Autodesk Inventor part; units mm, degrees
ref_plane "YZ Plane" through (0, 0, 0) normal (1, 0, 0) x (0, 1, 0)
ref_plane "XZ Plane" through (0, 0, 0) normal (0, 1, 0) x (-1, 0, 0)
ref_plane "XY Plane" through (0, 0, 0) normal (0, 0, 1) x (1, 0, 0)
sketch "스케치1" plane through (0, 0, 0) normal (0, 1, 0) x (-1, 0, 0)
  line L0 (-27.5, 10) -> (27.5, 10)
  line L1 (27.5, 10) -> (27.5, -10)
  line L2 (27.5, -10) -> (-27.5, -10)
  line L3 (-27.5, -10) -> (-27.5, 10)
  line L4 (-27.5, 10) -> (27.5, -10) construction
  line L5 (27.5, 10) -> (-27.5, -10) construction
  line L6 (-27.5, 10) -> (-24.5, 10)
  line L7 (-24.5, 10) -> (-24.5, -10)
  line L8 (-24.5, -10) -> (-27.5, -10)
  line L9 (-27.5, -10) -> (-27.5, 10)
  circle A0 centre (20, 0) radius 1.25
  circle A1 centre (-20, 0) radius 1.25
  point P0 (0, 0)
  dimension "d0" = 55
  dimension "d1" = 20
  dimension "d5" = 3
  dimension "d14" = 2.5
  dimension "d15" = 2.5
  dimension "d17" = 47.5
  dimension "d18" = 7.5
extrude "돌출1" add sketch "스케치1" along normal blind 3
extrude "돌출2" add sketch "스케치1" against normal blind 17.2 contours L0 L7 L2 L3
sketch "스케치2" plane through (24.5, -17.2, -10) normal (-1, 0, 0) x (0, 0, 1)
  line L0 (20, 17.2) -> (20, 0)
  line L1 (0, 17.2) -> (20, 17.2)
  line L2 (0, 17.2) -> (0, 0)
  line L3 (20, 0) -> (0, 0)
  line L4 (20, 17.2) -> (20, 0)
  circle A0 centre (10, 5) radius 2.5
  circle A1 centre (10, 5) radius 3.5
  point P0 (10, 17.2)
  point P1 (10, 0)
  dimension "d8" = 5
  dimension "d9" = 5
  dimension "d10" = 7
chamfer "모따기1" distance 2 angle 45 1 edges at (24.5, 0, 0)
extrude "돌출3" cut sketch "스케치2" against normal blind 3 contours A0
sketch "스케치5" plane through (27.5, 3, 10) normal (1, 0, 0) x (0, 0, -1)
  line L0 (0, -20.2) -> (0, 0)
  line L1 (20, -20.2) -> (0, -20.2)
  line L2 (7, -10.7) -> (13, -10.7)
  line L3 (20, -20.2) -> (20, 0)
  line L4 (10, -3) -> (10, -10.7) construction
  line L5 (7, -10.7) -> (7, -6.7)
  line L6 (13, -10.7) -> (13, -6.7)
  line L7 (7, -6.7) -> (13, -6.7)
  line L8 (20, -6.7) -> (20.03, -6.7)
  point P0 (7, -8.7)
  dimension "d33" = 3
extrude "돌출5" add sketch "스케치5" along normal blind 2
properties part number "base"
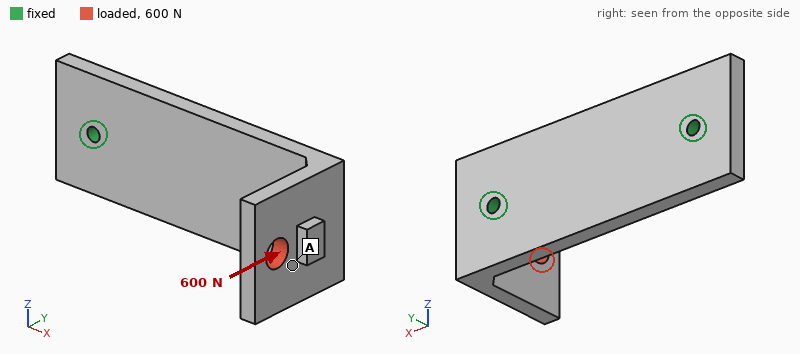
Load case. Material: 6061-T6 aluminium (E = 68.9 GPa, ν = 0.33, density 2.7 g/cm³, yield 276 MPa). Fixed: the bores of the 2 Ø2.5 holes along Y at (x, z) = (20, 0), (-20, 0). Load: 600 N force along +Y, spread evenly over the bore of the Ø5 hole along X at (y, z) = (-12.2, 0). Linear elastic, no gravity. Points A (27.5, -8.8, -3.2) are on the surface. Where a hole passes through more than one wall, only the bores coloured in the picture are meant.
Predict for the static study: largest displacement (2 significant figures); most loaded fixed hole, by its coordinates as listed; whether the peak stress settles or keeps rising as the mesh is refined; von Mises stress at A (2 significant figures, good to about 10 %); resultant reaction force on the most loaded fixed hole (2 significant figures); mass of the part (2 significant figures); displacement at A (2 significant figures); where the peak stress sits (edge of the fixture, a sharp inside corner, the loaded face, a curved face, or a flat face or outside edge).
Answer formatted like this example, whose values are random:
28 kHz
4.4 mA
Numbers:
88 µm
(20, 0)
keeps rising
22 MPa
620 N
12 g
55 µm
edge of the fixture
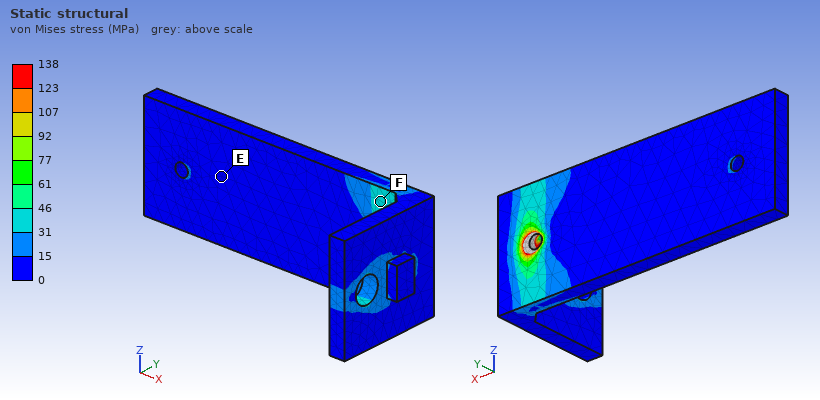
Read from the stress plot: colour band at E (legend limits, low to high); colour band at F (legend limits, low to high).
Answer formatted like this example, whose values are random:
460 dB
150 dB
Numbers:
0 to 15 MPa
31 to 46 MPa
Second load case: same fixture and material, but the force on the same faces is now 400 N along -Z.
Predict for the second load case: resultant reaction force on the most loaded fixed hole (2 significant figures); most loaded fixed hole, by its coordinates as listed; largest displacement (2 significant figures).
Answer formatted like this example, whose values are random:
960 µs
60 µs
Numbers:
450 N
(20, 0)
0.15 mm
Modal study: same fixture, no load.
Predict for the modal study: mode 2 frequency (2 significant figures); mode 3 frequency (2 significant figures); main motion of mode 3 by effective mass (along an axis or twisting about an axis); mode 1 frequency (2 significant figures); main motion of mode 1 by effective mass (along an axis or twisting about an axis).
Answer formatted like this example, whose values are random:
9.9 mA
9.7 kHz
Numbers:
6500 Hz
8500 Hz
along Y
5200 Hz
along X
